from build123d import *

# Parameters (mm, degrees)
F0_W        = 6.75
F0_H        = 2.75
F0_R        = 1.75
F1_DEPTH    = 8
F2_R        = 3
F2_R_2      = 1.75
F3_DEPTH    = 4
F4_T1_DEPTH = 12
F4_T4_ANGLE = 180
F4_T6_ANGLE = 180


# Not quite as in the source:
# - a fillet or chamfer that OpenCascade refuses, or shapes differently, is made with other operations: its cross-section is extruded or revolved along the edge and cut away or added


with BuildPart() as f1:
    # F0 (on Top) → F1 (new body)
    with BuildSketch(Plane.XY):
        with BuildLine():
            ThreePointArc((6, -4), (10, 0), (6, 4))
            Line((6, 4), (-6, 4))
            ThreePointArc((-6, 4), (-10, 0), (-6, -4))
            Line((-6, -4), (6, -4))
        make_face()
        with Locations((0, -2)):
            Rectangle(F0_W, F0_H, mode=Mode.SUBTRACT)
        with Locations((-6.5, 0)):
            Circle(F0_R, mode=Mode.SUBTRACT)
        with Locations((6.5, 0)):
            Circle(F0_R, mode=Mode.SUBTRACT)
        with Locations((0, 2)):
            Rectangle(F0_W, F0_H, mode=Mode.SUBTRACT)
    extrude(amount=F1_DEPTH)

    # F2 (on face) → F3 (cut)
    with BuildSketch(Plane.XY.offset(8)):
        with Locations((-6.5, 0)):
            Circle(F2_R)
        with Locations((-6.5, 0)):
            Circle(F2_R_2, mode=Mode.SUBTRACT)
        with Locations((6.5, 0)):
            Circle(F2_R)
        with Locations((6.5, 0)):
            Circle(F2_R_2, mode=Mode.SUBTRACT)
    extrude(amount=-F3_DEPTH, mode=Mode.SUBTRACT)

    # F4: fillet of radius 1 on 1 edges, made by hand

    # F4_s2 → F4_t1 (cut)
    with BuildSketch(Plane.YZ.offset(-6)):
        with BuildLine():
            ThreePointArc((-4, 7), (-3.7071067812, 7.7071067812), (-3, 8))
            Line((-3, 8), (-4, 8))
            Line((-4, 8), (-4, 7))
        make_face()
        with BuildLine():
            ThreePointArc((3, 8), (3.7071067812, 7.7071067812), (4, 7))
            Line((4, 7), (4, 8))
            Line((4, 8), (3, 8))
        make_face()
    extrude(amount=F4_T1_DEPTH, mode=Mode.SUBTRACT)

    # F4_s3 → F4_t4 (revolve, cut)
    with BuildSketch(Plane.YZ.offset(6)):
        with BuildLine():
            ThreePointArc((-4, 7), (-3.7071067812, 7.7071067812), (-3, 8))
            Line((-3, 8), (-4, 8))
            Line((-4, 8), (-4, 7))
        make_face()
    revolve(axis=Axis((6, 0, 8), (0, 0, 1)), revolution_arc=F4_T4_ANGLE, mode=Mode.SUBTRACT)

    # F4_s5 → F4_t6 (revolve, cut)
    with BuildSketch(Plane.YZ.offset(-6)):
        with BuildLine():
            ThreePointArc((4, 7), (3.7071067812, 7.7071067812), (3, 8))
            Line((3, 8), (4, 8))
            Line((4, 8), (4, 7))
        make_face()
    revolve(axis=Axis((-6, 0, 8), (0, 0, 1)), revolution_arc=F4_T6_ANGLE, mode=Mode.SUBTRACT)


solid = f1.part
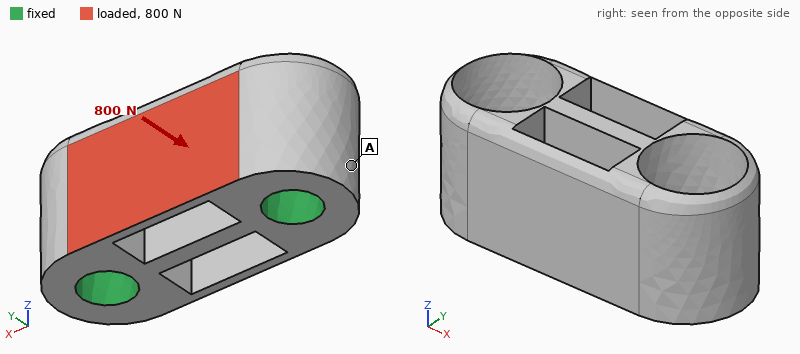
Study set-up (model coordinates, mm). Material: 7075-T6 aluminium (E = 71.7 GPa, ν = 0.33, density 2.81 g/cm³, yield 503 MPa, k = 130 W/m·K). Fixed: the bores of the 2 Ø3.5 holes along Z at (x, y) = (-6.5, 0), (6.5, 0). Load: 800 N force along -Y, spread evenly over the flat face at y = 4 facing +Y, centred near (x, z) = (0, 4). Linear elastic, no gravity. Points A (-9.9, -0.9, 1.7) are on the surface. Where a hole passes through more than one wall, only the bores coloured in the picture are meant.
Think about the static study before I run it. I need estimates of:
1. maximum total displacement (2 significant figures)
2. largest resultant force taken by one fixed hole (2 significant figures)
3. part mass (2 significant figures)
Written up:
54 µm
420 N
1.6 g
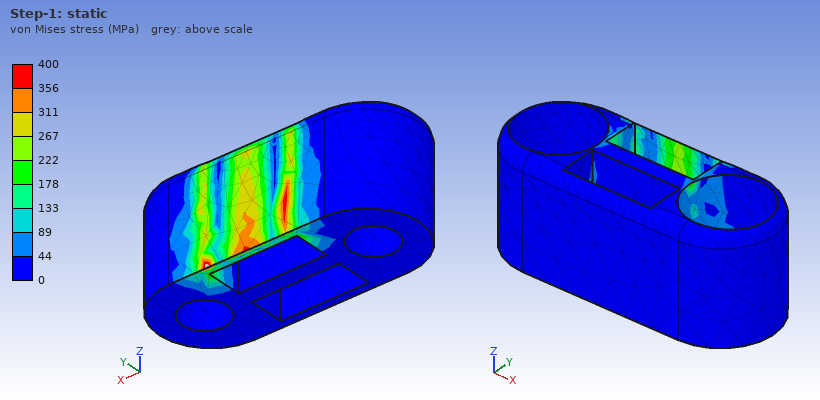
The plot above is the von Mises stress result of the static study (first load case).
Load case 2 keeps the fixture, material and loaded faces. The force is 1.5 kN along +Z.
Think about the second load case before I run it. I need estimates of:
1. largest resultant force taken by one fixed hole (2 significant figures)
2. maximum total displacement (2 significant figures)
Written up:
760 N
38 µm
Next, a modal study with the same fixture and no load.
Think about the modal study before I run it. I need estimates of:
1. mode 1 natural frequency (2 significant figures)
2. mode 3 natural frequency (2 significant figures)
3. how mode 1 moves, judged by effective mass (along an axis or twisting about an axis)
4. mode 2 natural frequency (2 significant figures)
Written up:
51 kHz
64 kHz
along Y
56 kHz
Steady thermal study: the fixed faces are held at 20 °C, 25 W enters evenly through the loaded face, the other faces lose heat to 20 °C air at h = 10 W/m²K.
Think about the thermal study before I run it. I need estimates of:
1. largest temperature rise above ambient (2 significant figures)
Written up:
42 K
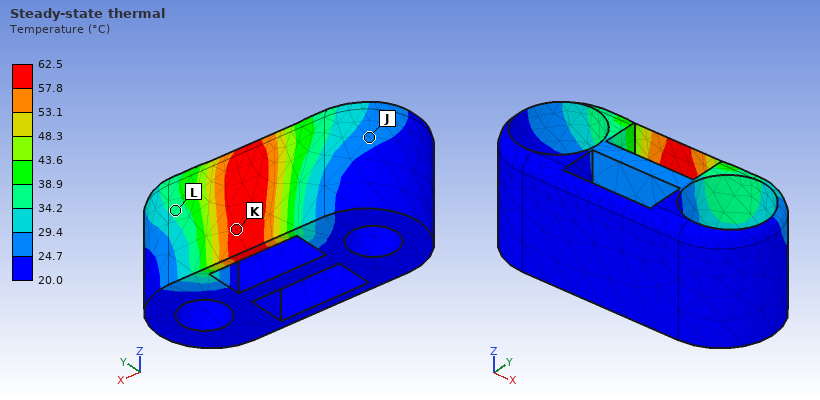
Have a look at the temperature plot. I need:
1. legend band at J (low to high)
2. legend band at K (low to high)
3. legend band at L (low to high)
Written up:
24.7 to 29.4 °C
57.8 to 62.5 °C
34.2 to 38.9 °C
